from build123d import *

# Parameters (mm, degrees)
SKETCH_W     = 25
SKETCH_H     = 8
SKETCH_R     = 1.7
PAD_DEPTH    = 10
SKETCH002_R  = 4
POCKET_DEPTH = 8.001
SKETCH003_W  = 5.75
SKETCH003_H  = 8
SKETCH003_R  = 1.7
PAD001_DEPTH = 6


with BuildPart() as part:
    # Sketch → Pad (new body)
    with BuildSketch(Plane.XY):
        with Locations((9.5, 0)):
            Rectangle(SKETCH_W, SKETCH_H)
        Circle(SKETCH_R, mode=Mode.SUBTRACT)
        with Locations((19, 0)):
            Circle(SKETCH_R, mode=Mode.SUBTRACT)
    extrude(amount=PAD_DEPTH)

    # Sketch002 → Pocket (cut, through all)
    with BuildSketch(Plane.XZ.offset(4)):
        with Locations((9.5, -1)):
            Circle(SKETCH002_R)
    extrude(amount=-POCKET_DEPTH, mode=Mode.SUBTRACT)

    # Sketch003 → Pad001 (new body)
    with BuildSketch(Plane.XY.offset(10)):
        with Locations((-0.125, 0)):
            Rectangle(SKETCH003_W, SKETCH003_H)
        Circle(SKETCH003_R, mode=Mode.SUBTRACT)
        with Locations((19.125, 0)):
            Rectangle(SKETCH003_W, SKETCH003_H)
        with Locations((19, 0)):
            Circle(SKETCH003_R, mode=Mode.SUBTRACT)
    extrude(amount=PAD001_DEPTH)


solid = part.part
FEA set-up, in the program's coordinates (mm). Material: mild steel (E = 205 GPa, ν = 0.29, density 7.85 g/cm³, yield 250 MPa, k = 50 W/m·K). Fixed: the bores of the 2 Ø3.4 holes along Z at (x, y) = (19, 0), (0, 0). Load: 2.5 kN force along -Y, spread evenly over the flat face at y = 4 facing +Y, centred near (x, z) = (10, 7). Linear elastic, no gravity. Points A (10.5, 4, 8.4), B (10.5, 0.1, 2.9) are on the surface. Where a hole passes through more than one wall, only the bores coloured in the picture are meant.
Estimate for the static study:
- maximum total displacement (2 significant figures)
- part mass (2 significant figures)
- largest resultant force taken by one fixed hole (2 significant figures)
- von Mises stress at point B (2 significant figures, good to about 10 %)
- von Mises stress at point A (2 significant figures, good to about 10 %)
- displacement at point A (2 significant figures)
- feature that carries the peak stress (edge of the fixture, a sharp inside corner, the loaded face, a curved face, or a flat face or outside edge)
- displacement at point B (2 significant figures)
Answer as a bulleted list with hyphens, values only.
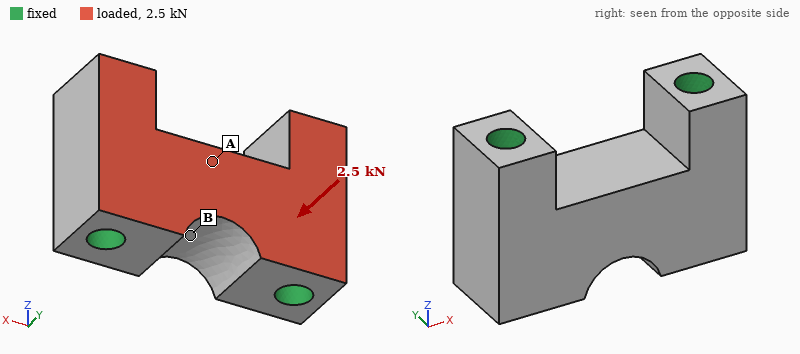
- 1.0 µm
- 17 g
- 1.3 kN
- 4.5 MPa
- 14 MPa
- 0.95 µm
- edge of the fixture
- 0.78 µm
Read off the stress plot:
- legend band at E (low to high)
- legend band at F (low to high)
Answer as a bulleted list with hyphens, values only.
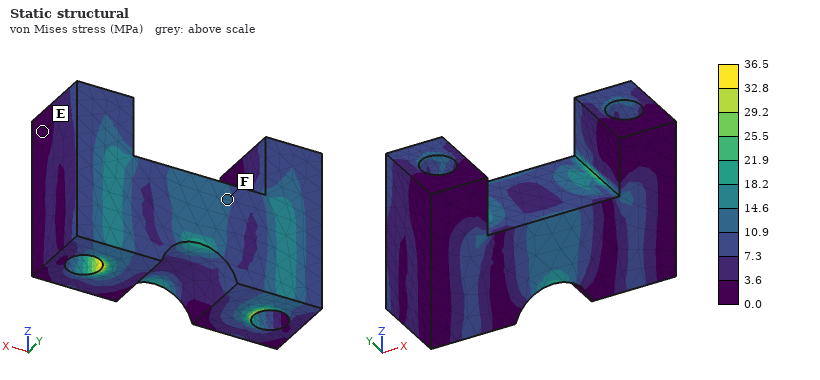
- 0.0 to 3.6 MPa
- 10.9 to 14.6 MPa
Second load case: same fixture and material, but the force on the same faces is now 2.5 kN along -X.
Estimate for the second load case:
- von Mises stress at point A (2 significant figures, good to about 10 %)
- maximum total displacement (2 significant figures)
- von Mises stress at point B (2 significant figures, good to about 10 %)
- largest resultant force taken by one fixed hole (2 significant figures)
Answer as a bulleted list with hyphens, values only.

- 14 MPa
- 0.73 µm
- 14 MPa
- 1.3 kN
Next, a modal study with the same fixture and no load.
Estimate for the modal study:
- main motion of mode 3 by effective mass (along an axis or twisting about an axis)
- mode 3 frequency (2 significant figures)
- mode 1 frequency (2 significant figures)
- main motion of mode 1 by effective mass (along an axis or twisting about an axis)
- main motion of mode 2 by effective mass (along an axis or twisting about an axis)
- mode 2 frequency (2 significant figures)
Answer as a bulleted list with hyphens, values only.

- twisting about X
- 100 kHz
- 70 kHz
- along Y
- along Z
- 84 kHz
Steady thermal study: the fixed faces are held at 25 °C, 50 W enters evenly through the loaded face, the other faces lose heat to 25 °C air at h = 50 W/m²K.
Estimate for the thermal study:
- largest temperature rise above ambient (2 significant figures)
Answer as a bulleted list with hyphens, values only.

- 23 K
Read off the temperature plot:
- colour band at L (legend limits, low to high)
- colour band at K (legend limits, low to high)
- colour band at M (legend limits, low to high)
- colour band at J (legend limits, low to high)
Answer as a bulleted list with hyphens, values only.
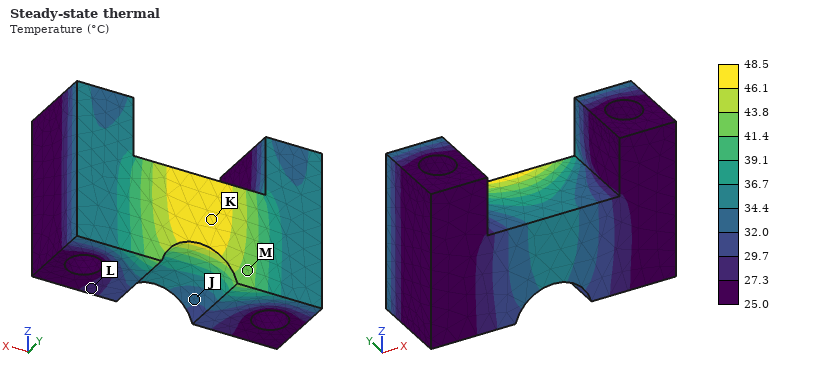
- 27.3 to 29.7 °C
- 46.1 to 48.5 °C
- 41.4 to 43.8 °C
- 32.0 to 34.4 °C
